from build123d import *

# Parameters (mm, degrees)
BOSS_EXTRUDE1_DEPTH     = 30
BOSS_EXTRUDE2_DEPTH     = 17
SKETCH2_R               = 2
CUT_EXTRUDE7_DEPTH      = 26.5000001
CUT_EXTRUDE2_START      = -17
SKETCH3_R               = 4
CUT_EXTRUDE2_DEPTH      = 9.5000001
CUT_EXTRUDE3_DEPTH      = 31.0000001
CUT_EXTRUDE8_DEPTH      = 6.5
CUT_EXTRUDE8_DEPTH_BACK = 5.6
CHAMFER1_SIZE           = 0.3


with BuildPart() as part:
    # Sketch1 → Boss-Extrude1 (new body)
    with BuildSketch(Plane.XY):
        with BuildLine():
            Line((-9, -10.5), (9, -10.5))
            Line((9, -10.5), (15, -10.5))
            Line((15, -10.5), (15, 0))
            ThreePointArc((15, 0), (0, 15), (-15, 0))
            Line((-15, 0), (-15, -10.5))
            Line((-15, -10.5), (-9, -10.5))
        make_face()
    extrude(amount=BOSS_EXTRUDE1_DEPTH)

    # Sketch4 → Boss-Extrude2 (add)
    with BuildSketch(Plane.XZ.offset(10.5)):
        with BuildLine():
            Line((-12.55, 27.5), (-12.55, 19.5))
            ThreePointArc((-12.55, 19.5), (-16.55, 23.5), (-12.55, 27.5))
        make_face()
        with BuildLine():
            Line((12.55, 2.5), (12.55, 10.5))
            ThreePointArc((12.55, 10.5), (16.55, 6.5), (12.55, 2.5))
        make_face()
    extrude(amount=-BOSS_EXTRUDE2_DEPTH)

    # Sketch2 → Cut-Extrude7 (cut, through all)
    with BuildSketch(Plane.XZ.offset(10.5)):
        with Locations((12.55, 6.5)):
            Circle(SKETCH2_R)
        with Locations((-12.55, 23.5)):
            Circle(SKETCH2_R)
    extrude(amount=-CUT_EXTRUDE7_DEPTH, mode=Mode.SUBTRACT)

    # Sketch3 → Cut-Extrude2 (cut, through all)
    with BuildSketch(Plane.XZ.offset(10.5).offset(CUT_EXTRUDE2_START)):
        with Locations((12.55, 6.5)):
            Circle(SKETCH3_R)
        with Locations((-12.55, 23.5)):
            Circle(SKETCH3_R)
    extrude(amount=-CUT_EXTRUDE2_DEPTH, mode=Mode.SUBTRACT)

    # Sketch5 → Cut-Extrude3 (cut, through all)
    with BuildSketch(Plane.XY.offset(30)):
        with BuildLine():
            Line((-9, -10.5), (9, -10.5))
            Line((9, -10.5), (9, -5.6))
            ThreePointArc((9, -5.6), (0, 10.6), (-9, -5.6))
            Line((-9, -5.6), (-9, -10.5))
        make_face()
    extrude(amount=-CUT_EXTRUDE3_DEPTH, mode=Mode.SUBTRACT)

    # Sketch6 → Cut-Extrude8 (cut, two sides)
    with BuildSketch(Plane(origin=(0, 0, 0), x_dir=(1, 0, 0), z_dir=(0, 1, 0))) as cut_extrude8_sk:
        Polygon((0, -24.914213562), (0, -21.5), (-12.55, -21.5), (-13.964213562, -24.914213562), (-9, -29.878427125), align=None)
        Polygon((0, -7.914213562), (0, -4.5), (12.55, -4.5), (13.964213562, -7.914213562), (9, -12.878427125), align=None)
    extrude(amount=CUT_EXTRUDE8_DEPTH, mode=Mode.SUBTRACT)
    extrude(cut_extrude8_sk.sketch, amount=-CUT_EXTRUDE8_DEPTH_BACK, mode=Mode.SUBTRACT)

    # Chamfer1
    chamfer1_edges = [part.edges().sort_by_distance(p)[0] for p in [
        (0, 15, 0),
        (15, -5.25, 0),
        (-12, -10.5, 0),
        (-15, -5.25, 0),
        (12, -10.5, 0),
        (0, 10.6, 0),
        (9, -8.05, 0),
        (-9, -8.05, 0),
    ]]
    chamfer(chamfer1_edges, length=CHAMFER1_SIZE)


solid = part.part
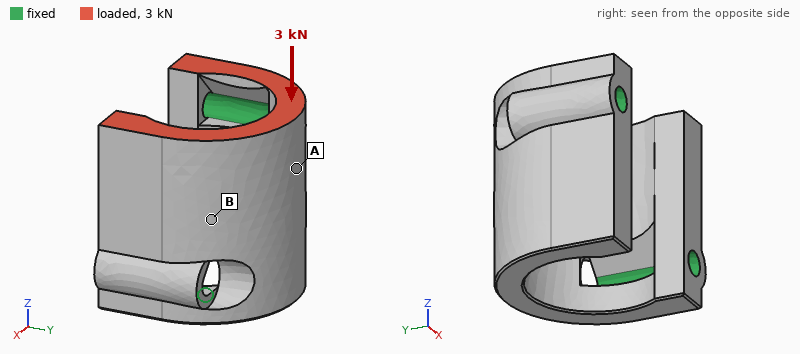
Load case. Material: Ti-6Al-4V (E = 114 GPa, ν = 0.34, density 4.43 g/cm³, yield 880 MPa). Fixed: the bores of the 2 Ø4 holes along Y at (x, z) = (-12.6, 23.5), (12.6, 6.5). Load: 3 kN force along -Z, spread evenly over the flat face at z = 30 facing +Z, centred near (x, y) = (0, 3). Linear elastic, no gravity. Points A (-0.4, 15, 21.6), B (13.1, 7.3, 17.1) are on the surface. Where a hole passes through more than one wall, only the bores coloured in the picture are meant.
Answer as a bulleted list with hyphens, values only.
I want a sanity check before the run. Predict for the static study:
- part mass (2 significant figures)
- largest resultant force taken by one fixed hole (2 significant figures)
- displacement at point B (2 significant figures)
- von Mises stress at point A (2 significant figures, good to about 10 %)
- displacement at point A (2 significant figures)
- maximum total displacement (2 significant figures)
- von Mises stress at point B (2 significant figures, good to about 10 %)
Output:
- 36 g
- 1.5 kN
- 9.3 µm
- 11 MPa
- 15 µm
- 19 µm
- 26 MPa
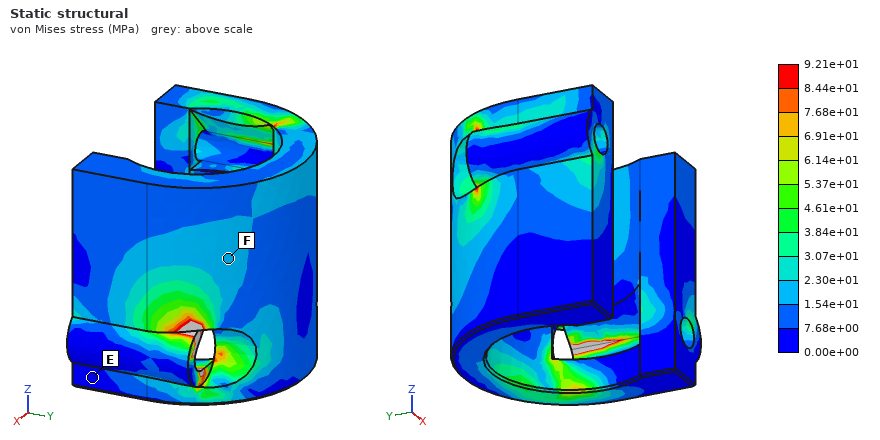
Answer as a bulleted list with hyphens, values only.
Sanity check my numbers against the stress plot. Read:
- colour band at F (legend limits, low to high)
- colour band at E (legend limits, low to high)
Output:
- 1.54e+01 to 2.30e+01 MPa
- 0.00e+00 to 7.68e+00 MPa
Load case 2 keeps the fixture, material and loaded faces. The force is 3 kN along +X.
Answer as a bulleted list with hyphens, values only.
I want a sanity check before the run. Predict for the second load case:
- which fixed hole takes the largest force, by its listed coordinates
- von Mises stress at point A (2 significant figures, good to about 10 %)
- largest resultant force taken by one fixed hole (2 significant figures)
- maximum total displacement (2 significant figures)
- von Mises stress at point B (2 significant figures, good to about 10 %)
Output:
- (-12.6, 23.5)
- 33 MPa
- 2.0 kN
- 90 µm
- 49 MPa
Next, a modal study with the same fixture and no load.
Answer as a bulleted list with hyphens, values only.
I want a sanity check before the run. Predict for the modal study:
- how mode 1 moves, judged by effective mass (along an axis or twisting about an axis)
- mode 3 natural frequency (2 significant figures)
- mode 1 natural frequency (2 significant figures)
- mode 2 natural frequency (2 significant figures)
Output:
- along X
- 14 kHz
- 9200 Hz
- 12 kHz
